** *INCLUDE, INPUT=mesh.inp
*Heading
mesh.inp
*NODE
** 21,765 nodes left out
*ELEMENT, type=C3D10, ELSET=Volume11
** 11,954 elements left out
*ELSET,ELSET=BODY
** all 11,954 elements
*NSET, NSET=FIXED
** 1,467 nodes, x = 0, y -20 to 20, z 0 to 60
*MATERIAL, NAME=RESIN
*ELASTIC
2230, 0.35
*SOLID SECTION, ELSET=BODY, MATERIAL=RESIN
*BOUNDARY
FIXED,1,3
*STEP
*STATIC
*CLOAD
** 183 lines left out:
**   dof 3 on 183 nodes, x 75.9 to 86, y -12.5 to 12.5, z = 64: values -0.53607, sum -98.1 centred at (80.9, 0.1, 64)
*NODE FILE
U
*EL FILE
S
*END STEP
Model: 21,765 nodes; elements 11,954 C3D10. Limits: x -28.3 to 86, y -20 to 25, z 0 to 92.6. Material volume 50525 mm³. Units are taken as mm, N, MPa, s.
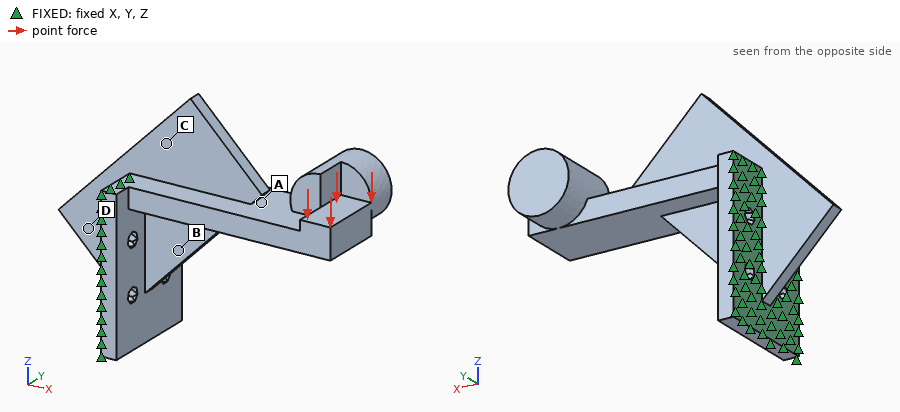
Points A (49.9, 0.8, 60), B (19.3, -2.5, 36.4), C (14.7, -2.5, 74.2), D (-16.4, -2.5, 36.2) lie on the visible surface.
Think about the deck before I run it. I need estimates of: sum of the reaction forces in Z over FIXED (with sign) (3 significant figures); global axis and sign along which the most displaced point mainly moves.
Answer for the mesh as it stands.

98.1 N
-Z
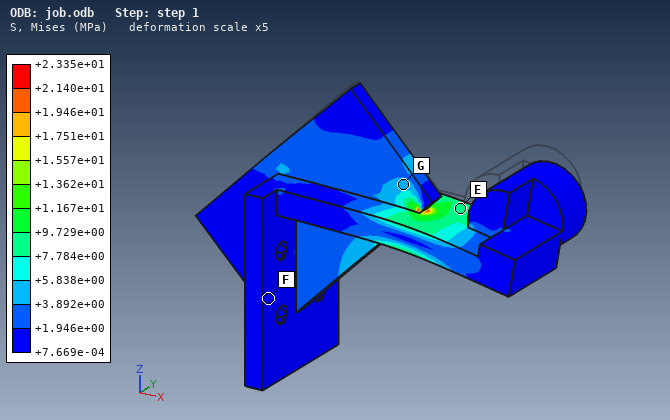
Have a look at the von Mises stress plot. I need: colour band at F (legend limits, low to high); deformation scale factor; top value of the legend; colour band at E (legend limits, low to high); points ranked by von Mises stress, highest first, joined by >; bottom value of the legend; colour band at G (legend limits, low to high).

+7.669e-04 to +1.946e+00 MPa
5
+2.335e+01 MPa
+7.784e+00 to +9.729e+00 MPa
E > G > F
+7.669e-04 MPa
+3.892e+00 to +5.838e+00 MPa
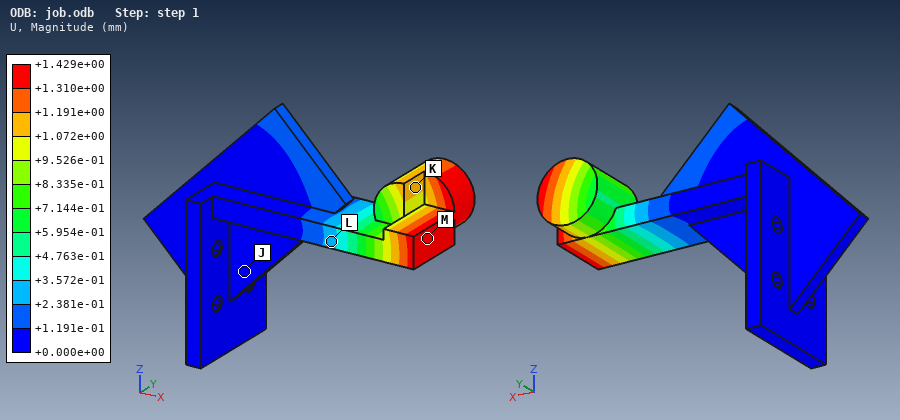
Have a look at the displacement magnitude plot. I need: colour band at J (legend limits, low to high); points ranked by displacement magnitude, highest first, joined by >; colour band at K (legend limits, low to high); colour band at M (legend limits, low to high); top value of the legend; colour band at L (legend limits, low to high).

+0.000e+00 to +1.191e-01 mm
M > K > L > J
+1.072e+00 to +1.191e+00 mm
+1.310e+00 to +1.429e+00 mm
+1.429e+00 mm
+2.381e-01 to +3.572e-01 mm
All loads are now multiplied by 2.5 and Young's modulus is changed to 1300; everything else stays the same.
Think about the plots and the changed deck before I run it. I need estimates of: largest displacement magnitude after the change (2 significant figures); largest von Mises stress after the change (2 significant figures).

6.1 mm
58 MPa
